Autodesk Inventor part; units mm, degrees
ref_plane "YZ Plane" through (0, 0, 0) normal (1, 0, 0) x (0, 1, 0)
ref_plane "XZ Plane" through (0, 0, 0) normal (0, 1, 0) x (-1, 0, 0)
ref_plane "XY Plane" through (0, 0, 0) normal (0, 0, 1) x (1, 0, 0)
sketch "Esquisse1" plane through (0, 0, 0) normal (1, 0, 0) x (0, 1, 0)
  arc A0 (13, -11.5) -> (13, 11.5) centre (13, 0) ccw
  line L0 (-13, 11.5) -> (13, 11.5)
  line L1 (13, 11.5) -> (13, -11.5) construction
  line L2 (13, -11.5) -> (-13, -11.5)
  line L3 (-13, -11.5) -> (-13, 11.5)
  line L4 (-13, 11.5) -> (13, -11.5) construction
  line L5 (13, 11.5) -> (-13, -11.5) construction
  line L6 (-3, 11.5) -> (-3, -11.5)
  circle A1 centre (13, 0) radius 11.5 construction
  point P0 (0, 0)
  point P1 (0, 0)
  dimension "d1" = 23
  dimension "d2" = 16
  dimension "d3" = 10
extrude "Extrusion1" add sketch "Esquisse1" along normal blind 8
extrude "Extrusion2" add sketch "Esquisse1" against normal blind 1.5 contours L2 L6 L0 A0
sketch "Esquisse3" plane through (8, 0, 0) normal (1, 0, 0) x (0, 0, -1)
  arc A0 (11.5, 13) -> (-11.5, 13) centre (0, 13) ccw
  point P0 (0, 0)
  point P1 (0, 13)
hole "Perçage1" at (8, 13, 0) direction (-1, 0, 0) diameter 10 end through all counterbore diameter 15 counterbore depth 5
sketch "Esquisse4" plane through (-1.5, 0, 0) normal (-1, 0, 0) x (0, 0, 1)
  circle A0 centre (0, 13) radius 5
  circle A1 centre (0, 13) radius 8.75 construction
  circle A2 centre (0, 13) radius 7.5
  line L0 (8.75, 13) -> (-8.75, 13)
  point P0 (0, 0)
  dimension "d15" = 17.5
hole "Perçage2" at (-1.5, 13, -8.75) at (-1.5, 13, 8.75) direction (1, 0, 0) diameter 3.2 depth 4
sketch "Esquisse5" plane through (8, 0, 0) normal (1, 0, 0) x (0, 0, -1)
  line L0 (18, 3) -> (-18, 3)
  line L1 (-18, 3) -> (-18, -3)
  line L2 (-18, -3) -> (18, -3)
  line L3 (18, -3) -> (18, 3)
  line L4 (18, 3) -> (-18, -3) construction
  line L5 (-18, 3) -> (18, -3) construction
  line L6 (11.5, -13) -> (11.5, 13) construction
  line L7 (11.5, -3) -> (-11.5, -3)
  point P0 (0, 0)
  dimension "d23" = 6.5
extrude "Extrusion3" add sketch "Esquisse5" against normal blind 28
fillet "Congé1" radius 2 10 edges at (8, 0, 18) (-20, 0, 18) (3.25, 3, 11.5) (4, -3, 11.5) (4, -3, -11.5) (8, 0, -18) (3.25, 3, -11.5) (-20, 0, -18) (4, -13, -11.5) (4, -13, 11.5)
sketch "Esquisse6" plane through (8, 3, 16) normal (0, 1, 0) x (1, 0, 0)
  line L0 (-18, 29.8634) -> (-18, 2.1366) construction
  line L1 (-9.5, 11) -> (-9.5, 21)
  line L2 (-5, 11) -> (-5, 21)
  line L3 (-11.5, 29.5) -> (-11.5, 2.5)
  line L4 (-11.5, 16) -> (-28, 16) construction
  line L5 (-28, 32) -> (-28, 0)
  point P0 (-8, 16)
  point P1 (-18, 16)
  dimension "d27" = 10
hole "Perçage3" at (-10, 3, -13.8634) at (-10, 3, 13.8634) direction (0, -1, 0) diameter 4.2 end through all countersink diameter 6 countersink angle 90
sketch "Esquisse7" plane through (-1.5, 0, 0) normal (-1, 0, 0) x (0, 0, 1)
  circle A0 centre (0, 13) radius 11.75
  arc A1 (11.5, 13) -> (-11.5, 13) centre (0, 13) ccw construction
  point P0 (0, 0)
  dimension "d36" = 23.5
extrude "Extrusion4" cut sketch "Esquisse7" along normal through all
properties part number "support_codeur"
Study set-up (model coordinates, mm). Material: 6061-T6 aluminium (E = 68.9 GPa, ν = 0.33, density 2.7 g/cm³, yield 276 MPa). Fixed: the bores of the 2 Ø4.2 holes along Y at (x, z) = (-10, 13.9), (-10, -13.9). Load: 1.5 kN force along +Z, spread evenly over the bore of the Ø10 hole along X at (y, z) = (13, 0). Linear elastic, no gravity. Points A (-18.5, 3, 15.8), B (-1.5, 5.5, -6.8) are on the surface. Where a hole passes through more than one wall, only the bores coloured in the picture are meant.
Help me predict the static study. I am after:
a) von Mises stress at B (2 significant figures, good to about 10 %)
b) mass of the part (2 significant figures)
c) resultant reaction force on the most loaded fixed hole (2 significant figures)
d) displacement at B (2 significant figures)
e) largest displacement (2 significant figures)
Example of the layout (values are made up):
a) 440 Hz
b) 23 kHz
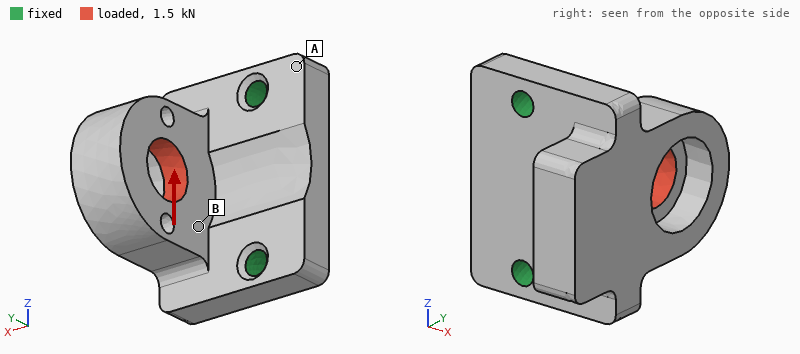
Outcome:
a) 30 MPa
b) 28 g
c) 1.2 kN
d) 13 µm
e) 48 µm
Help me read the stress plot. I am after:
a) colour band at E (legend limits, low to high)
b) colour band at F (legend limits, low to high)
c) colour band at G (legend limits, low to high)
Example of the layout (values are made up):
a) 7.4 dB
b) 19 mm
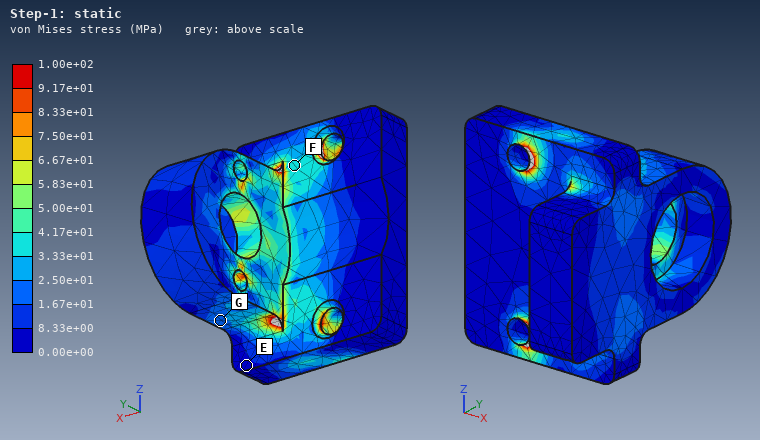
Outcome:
a) 0.00e+00 to 8.33e+00 MPa
b) 3.33e+01 to 4.17e+01 MPa
c) 1.67e+01 to 2.50e+01 MPa
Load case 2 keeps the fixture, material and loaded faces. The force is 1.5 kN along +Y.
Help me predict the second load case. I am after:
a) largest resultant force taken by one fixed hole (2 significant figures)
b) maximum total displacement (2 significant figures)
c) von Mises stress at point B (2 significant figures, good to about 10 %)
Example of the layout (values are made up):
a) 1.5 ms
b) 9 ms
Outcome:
a) 750 N
b) 71 µm
c) 19 MPa
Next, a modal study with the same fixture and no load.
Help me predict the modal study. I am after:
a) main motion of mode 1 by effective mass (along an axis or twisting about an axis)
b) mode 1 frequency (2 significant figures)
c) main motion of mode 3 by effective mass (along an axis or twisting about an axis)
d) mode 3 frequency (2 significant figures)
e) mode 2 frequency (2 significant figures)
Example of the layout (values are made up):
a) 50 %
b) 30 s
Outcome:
a) along Y
b) 4700 Hz
c) along Y
d) 13 kHz
e) 11 kHz
